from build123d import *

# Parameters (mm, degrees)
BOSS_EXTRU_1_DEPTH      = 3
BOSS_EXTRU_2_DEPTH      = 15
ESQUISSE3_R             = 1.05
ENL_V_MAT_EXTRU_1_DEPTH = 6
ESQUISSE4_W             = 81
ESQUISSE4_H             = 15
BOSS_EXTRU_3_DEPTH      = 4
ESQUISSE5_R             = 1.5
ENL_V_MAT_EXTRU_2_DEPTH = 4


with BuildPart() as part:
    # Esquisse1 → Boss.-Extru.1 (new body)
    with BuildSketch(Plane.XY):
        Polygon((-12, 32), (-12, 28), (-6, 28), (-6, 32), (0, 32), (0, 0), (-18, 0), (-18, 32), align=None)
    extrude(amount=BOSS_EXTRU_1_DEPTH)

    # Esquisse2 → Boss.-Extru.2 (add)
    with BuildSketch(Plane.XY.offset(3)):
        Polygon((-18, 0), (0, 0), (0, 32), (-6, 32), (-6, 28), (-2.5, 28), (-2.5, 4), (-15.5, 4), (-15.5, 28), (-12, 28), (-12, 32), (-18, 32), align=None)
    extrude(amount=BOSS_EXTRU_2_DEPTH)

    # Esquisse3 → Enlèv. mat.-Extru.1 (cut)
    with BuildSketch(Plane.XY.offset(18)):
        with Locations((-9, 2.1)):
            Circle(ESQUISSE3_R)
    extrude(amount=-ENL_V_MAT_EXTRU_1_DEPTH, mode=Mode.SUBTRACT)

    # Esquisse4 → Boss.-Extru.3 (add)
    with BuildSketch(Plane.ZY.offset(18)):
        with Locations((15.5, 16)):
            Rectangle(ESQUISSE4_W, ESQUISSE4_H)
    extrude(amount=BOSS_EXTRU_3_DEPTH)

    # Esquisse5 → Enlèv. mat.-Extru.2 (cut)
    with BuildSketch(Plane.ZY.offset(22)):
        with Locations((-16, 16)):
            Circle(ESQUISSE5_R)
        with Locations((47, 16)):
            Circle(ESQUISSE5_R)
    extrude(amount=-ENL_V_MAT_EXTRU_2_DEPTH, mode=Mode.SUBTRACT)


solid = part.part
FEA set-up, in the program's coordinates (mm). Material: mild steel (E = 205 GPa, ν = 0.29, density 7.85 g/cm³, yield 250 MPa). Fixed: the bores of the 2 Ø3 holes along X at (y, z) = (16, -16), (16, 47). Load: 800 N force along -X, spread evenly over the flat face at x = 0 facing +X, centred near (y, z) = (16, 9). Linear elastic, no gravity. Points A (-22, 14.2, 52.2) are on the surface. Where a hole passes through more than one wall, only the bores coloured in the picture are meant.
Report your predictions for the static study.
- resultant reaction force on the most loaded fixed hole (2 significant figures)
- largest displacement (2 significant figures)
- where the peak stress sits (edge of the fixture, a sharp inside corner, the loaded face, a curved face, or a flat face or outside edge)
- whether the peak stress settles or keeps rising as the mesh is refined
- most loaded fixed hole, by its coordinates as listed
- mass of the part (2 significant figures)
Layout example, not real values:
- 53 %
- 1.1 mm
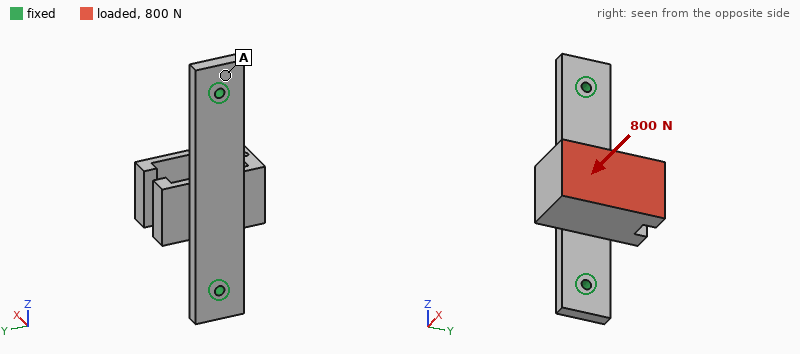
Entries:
- 570 N
- 0.11 mm
- edge of the fixture
- keeps rising
- (16, -16)
- 79 g
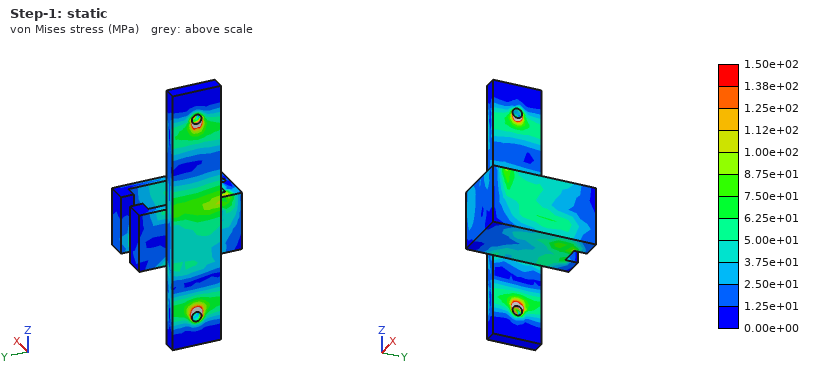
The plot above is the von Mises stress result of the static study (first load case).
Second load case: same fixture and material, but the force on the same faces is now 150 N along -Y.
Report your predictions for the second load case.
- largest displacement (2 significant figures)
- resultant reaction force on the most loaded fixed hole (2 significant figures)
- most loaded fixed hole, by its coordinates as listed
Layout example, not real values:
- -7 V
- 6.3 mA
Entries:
- 41 µm
- 93 N
- (16, -16)
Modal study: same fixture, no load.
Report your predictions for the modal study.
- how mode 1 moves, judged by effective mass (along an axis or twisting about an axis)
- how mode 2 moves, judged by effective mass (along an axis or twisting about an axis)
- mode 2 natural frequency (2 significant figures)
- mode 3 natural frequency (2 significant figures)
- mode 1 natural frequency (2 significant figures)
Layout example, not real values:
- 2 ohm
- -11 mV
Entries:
- along Y
- along X
- 2800 Hz
- 4900 Hz
- 2100 Hz
